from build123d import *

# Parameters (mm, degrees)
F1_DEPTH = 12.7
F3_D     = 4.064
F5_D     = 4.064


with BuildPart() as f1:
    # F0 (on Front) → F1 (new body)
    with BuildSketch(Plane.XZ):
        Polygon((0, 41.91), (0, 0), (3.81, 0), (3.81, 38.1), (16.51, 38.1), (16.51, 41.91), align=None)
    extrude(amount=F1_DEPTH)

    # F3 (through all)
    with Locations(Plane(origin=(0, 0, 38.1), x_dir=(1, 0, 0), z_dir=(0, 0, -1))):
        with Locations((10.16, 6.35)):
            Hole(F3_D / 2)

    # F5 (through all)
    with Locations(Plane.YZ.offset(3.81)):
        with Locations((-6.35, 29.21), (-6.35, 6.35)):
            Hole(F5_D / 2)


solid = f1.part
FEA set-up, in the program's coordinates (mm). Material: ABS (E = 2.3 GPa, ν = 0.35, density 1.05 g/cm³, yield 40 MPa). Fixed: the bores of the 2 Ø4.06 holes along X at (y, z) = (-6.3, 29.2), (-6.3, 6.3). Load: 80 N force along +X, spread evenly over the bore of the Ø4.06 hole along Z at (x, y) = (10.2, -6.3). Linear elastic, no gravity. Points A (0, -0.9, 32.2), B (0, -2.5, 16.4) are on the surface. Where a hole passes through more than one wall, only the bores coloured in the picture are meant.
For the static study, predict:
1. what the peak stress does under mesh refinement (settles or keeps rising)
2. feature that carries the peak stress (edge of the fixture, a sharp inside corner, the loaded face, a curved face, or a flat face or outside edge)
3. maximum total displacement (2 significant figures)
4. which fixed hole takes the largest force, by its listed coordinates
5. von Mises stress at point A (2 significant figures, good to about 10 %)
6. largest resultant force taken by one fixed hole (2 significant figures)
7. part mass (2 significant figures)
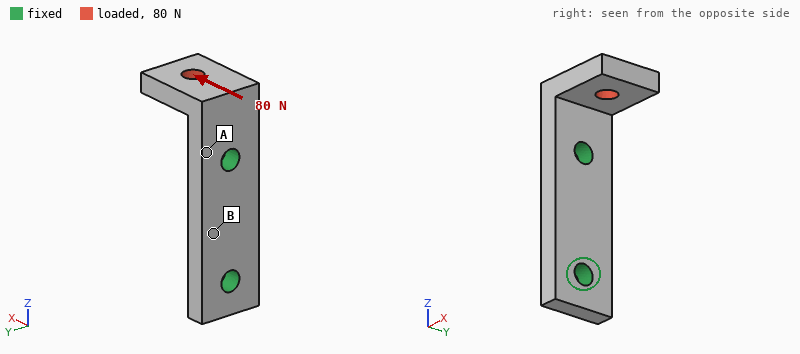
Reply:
keeps rising
edge of the fixture
0.51 mm
(-6.3, 29.2)
13 MPa
83 N
2.6 g
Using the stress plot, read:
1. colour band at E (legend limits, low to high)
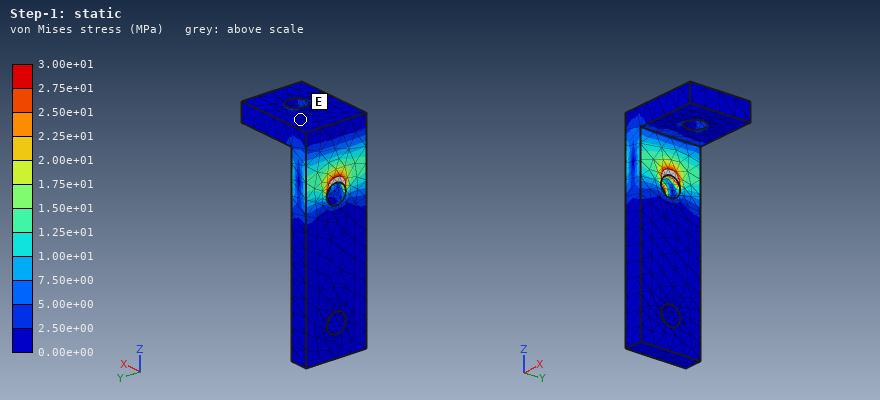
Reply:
0.00e+00 to 2.50e+00 MPa
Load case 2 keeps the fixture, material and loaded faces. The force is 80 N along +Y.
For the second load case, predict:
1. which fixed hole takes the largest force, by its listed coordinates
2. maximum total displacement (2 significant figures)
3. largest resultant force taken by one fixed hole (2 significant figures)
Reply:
(-6.3, 29.2)
0.56 mm
97 N
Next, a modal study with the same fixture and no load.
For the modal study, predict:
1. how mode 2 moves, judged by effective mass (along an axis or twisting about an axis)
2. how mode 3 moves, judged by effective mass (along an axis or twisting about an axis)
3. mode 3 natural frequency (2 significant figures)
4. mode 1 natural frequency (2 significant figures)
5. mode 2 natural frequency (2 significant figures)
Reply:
along Y
along X
5600 Hz
2100 Hz
2800 Hz
